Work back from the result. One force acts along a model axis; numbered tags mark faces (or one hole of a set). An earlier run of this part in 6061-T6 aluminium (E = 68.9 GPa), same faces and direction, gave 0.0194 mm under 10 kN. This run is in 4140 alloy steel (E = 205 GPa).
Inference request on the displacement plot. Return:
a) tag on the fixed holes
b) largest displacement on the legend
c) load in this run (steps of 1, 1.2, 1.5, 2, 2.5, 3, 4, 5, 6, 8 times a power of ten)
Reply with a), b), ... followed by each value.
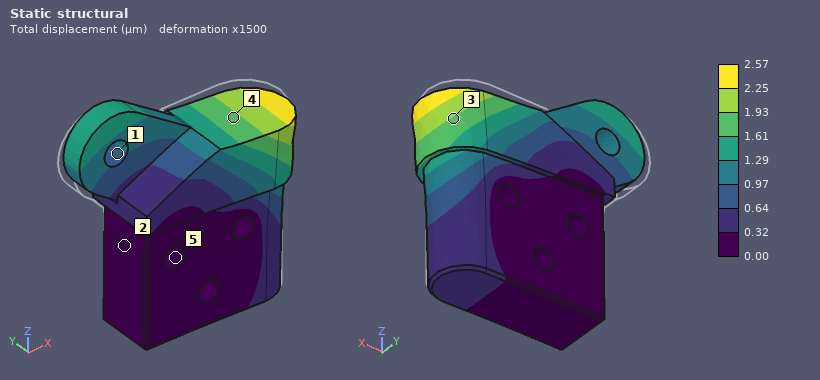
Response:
a) 5
b) 2.57 µm
c) 4 kN
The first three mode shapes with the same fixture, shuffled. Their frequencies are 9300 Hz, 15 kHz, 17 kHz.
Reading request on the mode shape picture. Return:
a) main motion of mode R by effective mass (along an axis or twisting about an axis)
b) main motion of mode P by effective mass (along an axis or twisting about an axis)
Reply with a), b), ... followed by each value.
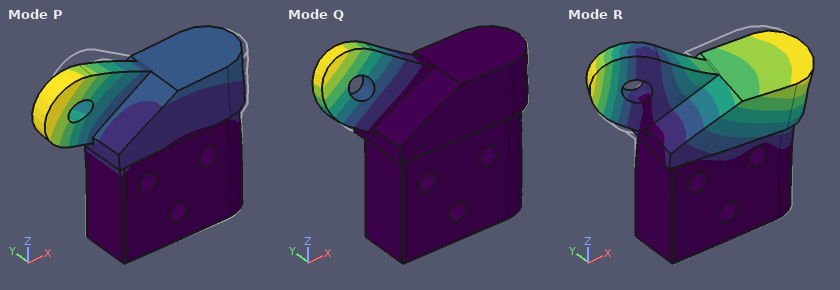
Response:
a) along Y
b) along X
